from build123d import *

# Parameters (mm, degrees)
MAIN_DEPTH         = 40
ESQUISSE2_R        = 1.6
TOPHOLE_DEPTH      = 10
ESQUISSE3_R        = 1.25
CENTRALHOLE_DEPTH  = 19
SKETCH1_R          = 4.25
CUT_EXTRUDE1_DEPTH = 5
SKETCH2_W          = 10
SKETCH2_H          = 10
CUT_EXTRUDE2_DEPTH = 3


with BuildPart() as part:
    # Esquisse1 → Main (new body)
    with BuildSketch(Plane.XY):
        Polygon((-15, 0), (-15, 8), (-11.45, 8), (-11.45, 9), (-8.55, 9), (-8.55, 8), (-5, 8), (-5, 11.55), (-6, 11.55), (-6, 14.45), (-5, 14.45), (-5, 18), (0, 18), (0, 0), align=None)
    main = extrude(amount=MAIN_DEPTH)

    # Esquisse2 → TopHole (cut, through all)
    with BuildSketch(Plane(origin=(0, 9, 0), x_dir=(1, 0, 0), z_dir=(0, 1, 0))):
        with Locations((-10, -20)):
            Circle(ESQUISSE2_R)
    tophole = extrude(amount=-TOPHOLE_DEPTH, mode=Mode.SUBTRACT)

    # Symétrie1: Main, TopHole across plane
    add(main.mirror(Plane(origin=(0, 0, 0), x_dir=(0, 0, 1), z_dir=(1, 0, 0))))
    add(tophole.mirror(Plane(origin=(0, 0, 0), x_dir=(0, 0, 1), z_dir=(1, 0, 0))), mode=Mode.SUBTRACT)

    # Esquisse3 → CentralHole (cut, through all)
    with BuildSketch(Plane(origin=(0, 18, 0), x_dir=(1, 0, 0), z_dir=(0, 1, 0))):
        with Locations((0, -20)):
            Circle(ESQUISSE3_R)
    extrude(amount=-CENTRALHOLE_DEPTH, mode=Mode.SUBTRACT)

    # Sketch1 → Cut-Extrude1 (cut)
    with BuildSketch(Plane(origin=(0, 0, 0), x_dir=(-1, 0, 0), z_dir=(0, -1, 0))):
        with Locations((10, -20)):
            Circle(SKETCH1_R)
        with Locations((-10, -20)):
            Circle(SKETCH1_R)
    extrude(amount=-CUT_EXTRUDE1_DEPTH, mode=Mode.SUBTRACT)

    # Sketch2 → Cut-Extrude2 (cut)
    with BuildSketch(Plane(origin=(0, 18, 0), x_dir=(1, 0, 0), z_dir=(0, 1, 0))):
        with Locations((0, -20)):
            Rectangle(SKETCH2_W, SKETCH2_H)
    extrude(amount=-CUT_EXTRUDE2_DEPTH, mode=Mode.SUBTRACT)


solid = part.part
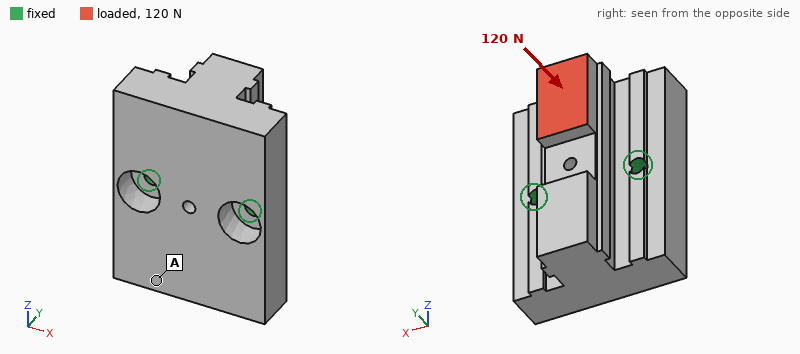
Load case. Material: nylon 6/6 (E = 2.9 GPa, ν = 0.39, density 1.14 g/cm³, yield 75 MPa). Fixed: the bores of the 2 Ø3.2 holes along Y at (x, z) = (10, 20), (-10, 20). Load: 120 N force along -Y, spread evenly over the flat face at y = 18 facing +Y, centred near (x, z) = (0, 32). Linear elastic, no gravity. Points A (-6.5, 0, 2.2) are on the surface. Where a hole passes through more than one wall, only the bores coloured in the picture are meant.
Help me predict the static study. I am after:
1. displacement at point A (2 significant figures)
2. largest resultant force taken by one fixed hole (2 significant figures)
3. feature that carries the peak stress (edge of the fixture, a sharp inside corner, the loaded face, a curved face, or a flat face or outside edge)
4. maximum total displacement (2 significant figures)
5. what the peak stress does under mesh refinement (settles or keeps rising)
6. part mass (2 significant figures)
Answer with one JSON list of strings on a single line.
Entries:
["0.13 mm", "60 N", "edge of the fixture", "0.20 mm", "keeps rising", "15 g"]
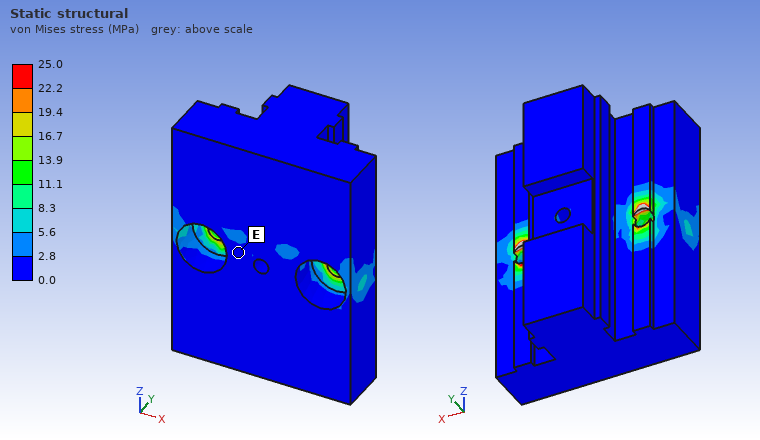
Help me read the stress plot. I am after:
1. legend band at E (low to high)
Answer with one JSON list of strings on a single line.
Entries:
["0.0 to 2.8 MPa"]
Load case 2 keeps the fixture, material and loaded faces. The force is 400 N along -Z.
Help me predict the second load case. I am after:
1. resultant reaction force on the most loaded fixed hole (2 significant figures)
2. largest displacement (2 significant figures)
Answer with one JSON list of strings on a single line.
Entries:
["200 N", "0.64 mm"]
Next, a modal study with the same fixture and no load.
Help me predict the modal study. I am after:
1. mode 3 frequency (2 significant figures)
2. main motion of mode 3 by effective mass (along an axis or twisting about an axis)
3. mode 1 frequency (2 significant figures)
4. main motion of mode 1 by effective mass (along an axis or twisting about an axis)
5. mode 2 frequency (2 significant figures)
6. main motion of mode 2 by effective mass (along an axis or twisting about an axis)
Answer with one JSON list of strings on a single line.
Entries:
["5000 Hz", "twisting about Y", "1400 Hz", "twisting about X", "4100 Hz", "along Y"]
